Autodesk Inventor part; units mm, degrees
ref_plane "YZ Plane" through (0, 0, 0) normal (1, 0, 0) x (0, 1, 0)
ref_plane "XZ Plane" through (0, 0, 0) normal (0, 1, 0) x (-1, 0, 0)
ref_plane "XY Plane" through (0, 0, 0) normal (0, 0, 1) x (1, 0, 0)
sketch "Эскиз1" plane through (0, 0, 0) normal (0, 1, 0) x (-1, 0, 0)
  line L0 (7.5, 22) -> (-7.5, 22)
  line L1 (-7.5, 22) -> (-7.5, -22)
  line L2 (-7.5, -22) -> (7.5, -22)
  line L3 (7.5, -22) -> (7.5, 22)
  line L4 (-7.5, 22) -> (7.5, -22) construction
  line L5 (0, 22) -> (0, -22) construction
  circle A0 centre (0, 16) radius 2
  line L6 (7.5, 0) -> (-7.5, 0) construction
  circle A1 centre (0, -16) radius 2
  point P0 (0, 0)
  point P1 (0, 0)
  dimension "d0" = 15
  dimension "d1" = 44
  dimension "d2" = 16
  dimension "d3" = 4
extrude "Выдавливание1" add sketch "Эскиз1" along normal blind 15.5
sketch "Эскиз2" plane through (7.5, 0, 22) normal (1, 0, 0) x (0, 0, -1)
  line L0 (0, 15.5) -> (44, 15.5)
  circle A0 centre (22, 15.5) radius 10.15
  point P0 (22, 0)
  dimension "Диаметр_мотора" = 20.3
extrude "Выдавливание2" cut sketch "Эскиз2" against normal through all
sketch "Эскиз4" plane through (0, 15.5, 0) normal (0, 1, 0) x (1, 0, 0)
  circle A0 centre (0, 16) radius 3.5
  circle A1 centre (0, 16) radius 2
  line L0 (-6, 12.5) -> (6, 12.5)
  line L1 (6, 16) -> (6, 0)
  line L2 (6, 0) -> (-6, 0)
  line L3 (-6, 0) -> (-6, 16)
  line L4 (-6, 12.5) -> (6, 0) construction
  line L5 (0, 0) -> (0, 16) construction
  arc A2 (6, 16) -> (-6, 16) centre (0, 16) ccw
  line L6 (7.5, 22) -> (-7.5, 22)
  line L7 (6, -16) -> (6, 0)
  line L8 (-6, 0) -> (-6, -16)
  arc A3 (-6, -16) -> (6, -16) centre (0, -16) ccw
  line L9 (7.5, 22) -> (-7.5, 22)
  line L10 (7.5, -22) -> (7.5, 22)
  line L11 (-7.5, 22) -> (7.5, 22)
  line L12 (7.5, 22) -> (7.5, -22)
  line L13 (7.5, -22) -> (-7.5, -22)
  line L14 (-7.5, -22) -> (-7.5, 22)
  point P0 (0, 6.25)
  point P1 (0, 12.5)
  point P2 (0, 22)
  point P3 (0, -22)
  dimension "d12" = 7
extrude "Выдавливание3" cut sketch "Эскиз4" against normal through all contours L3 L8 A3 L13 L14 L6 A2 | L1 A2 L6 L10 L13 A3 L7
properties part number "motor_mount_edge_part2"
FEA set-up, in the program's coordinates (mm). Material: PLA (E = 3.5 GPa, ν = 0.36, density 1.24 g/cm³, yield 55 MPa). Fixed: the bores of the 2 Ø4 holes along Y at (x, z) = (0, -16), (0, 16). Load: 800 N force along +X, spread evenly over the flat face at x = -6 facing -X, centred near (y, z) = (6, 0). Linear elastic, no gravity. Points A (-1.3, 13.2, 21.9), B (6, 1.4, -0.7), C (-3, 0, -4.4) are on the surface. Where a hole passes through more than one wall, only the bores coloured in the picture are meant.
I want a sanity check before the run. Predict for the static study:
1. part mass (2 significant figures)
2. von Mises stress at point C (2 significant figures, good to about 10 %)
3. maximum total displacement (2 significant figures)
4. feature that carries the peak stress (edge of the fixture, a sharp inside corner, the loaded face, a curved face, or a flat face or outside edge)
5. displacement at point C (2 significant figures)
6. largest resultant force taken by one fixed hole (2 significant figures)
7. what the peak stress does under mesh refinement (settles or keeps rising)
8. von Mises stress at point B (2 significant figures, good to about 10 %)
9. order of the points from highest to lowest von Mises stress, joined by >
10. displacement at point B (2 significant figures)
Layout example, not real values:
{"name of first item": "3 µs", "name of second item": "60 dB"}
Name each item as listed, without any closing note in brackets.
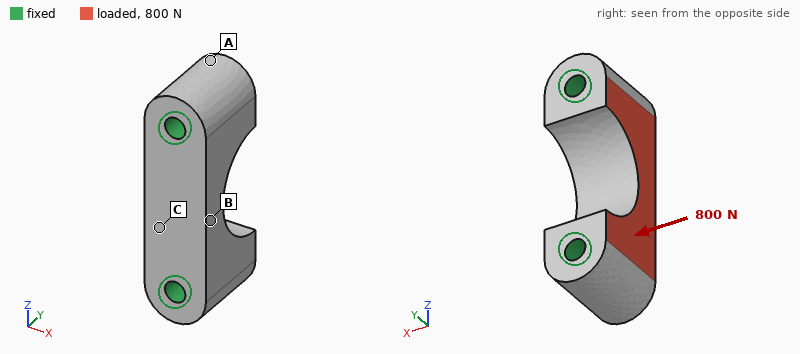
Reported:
{"part mass": "6.7 g", "von Mises stress at point C": "3.3 MPa", "maximum total displacement": "44 µm", "feature that carries the peak stress": "edge of the fixture", "displacement at point C": "37 µm", "largest resultant force taken by one fixed hole": "400 N", "what the peak stress does under mesh refinement": "keeps rising", "von Mises stress at point B": "5.8 MPa", "order of the points from highest to lowest von Mises stress, joined by >": "B > C > A", "displacement at point B": "37 µm"}
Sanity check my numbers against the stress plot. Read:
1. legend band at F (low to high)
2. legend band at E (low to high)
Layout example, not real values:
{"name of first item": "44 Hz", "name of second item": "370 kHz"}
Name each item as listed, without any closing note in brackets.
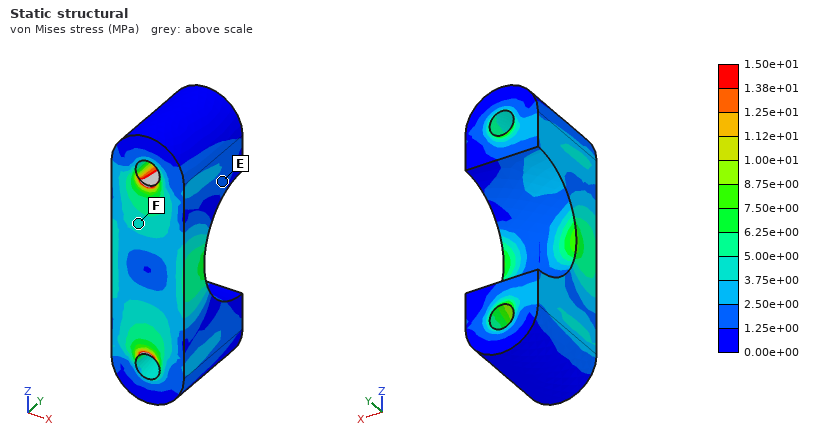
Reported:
{"legend band at F": "3.75e+00 to 5.00e+00 MPa", "legend band at E": "1.25e+00 to 2.50e+00 MPa"}
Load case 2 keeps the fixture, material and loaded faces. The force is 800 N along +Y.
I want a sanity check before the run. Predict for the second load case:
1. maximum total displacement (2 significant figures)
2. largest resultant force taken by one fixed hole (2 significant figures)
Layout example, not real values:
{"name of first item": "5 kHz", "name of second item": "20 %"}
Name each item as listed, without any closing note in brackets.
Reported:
{"maximum total displacement": "67 µm", "largest resultant force taken by one fixed hole": "410 N"}
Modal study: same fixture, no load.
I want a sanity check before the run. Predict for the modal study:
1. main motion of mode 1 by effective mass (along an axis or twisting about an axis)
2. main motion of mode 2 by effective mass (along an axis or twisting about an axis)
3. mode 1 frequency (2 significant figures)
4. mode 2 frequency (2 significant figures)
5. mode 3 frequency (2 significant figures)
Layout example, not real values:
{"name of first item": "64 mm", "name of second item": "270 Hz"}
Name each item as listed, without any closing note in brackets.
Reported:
{"main motion of mode 1 by effective mass": "along X", "main motion of mode 2 by effective mass": "along Y", "mode 1 frequency": "12 kHz", "mode 2 frequency": "16 kHz", "mode 3 frequency": "22 kHz"}
